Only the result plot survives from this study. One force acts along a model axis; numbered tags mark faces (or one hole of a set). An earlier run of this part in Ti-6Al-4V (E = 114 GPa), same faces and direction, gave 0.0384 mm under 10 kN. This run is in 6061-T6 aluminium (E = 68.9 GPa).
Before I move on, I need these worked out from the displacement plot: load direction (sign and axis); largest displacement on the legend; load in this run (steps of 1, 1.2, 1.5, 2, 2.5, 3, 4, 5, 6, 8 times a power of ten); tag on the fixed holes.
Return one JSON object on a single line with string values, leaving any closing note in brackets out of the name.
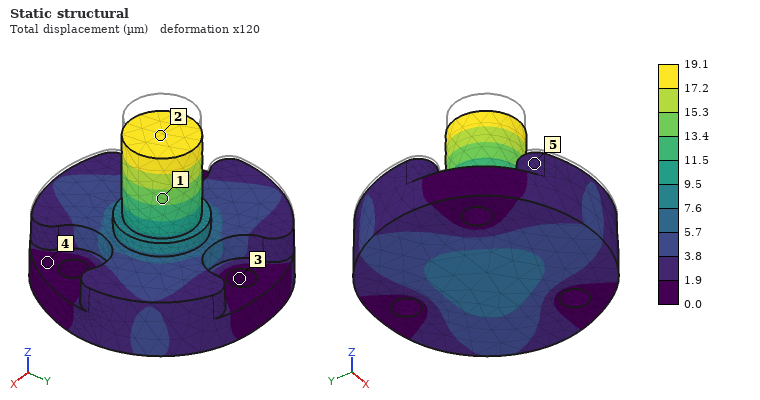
{"load direction": "-Z", "largest displacement on the legend": "19.1 µm", "load in this run": "3 kN", "tag on the fixed holes": "3"}
